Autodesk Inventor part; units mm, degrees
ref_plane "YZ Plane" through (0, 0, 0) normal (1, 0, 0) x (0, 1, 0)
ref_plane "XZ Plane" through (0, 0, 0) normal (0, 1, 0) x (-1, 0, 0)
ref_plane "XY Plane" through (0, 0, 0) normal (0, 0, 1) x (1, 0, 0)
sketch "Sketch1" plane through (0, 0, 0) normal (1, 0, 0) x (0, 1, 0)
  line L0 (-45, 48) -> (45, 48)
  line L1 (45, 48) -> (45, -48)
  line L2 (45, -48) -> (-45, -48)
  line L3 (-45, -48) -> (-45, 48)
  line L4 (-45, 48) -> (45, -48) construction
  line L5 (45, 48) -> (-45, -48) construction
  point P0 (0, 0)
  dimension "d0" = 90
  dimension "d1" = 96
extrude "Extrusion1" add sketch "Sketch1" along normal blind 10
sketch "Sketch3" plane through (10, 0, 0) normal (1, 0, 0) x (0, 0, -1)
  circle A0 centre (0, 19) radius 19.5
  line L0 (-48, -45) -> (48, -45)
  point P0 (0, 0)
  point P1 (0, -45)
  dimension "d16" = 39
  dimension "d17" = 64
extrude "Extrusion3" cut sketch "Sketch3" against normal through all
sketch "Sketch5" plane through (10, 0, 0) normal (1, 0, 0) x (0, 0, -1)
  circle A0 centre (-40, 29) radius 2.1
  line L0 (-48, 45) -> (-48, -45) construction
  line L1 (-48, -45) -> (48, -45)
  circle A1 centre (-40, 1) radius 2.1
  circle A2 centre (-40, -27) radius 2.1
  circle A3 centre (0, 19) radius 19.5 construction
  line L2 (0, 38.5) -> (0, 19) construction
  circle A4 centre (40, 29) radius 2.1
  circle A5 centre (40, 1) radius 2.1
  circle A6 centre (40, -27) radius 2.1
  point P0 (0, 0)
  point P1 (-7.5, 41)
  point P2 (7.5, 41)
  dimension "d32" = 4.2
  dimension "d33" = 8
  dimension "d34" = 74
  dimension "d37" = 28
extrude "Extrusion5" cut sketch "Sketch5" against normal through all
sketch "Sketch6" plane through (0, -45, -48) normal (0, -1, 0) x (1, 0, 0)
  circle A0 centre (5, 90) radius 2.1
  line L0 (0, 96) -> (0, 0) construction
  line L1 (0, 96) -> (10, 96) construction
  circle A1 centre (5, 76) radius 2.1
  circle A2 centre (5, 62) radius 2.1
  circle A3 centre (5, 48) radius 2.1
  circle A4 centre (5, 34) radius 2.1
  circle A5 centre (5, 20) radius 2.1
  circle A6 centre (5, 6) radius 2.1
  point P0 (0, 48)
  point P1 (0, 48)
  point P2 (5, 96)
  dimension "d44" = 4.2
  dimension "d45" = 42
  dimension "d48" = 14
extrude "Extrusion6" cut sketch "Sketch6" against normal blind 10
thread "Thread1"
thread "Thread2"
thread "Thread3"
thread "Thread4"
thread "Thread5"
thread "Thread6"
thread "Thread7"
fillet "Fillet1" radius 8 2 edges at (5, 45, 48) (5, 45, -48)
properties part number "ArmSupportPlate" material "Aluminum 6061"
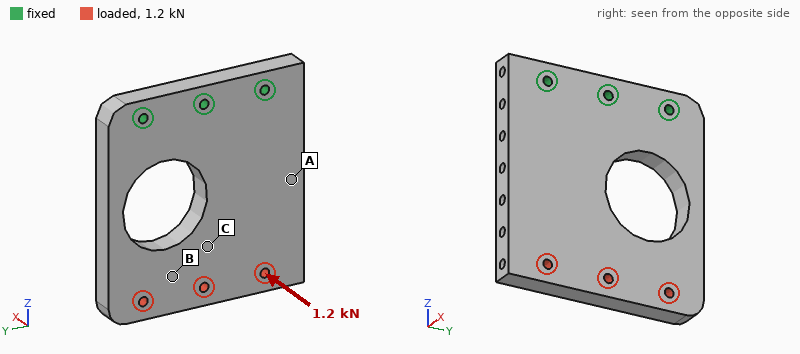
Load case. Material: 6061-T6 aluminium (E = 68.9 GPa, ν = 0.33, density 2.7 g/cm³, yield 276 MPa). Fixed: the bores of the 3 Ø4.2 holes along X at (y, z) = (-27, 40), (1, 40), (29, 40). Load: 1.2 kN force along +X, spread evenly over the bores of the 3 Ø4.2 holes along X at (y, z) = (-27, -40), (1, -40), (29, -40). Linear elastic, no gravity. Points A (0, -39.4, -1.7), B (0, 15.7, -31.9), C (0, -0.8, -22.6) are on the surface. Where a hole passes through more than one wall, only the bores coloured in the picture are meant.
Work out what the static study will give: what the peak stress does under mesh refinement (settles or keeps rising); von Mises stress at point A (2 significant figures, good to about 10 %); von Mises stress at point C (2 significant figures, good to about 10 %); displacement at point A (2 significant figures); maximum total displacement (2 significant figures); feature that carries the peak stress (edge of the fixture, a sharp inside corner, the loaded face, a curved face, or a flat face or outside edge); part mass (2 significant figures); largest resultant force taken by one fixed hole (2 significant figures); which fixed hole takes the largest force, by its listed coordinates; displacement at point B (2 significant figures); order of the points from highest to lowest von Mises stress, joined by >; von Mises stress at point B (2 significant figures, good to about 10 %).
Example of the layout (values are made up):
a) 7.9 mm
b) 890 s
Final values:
a) keeps rising
b) 43 MPa
c) 21 MPa
d) 0.20 mm
e) 0.71 mm
f) edge of the fixture
g) 200 g
h) 660 N
i) (1, 40)
j) 0.52 mm
k) A > C > B
l) 11 MPa
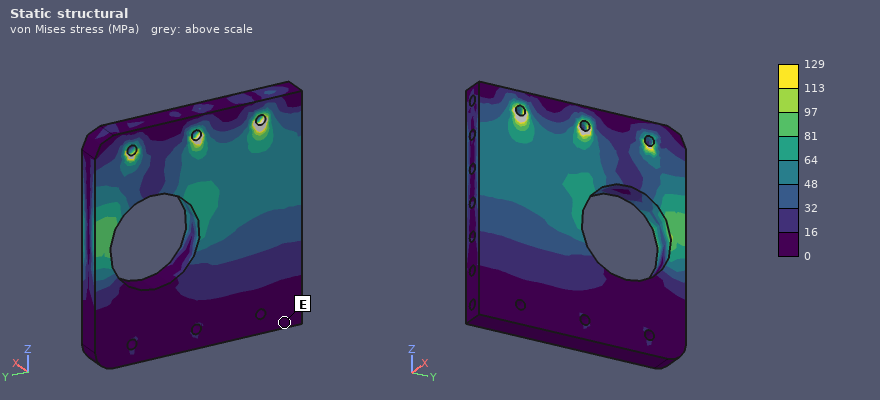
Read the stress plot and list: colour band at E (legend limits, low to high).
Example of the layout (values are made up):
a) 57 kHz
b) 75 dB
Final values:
a) 0 to 16 MPa
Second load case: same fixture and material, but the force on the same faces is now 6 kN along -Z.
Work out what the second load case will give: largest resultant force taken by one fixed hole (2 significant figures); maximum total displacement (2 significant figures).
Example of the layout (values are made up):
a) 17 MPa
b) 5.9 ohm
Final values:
a) 2.3 kN
b) 28 µm
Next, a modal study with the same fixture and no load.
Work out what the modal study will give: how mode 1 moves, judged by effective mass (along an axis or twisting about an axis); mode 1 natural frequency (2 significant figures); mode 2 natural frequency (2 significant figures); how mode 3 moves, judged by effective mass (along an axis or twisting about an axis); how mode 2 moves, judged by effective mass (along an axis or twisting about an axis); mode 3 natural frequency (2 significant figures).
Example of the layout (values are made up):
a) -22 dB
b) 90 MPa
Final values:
a) along X
b) 910 Hz
c) 2100 Hz
d) along Y
e) twisting about Z
f) 4000 Hz
